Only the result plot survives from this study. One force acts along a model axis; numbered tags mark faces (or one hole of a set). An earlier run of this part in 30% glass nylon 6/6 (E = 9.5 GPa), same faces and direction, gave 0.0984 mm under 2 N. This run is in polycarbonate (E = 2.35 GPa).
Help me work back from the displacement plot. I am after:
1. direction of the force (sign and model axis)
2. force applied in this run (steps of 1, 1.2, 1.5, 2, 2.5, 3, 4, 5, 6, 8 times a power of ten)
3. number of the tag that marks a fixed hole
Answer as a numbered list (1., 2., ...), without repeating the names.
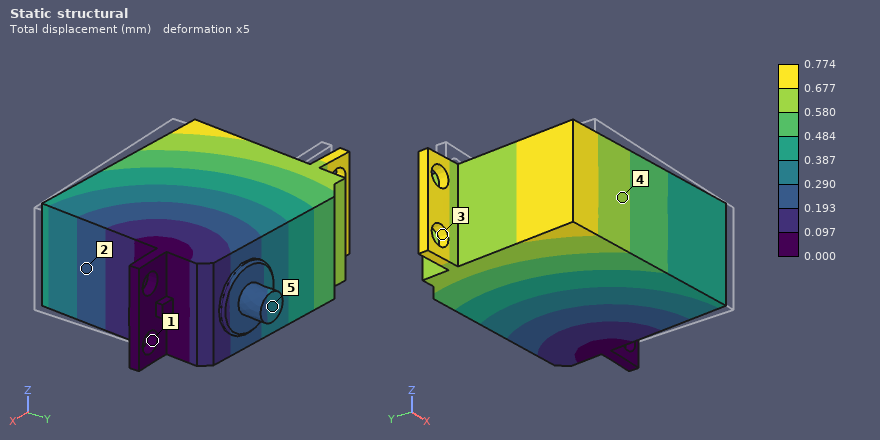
1. +Y
2. 4 N
3. 1
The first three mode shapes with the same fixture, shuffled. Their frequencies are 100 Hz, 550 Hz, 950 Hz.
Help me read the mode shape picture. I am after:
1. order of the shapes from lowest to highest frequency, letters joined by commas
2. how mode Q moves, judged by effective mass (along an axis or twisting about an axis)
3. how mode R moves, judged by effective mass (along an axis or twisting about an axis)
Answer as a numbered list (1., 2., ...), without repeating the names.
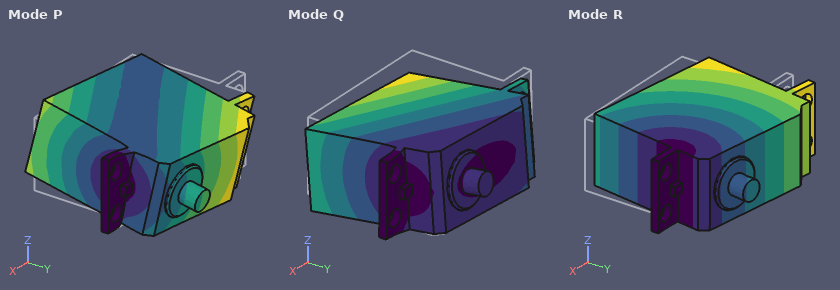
1. R, Q, P
2. along Z
3. along Y
